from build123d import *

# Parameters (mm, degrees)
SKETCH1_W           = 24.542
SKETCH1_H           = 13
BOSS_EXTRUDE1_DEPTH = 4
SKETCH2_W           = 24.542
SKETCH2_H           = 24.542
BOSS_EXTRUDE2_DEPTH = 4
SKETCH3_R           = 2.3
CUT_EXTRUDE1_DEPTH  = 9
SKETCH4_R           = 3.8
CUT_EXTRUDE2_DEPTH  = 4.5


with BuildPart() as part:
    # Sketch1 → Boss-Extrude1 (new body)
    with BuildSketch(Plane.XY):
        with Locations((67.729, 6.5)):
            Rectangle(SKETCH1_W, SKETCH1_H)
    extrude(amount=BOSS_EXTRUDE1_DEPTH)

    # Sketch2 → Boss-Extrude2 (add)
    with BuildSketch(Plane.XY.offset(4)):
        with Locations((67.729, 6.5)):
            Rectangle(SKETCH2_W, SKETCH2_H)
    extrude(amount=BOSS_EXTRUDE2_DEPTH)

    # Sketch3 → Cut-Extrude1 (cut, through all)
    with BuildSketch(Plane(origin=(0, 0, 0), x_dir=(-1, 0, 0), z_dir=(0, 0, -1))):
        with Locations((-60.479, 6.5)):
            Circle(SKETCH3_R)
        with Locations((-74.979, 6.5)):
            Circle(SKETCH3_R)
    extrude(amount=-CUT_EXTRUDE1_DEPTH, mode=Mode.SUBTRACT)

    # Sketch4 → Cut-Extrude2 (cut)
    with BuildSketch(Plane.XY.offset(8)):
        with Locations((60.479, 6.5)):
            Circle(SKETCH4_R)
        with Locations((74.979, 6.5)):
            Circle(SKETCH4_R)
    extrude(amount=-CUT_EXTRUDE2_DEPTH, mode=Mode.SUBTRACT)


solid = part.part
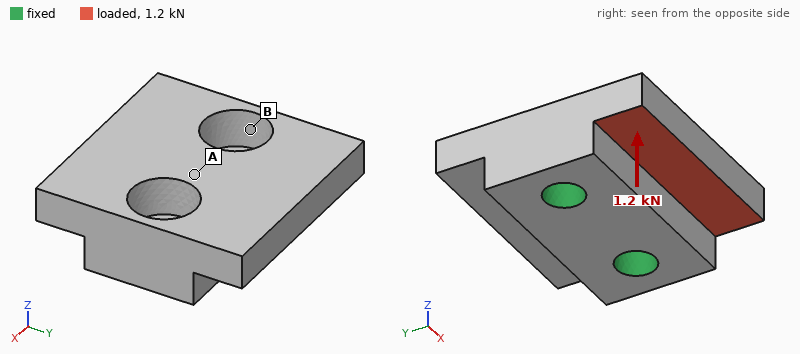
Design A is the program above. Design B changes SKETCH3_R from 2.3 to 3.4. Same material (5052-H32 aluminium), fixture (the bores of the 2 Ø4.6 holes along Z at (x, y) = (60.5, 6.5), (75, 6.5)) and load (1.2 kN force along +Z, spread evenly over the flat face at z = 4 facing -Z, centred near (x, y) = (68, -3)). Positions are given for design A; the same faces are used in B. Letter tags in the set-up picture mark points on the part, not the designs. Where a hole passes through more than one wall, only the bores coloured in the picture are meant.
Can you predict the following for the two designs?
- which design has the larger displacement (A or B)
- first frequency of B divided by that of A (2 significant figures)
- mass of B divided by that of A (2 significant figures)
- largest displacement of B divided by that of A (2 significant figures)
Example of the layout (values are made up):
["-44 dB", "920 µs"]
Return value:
["A", "1.4", "0.96", "0.68"]
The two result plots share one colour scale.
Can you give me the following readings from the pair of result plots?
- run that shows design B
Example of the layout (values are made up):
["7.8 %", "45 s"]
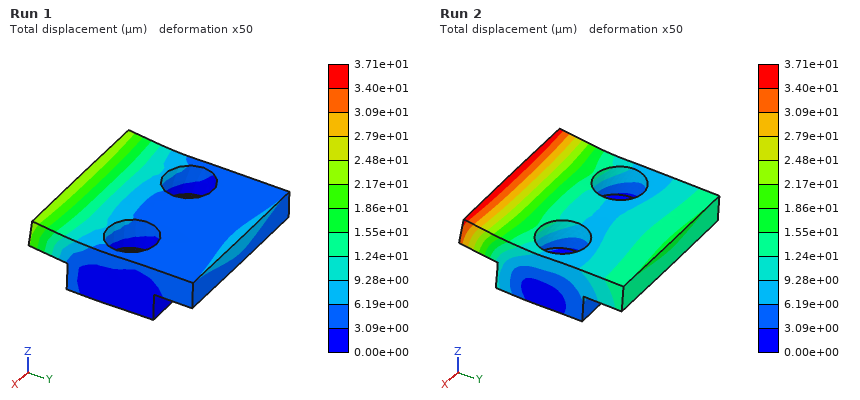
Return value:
["Run 1"]
